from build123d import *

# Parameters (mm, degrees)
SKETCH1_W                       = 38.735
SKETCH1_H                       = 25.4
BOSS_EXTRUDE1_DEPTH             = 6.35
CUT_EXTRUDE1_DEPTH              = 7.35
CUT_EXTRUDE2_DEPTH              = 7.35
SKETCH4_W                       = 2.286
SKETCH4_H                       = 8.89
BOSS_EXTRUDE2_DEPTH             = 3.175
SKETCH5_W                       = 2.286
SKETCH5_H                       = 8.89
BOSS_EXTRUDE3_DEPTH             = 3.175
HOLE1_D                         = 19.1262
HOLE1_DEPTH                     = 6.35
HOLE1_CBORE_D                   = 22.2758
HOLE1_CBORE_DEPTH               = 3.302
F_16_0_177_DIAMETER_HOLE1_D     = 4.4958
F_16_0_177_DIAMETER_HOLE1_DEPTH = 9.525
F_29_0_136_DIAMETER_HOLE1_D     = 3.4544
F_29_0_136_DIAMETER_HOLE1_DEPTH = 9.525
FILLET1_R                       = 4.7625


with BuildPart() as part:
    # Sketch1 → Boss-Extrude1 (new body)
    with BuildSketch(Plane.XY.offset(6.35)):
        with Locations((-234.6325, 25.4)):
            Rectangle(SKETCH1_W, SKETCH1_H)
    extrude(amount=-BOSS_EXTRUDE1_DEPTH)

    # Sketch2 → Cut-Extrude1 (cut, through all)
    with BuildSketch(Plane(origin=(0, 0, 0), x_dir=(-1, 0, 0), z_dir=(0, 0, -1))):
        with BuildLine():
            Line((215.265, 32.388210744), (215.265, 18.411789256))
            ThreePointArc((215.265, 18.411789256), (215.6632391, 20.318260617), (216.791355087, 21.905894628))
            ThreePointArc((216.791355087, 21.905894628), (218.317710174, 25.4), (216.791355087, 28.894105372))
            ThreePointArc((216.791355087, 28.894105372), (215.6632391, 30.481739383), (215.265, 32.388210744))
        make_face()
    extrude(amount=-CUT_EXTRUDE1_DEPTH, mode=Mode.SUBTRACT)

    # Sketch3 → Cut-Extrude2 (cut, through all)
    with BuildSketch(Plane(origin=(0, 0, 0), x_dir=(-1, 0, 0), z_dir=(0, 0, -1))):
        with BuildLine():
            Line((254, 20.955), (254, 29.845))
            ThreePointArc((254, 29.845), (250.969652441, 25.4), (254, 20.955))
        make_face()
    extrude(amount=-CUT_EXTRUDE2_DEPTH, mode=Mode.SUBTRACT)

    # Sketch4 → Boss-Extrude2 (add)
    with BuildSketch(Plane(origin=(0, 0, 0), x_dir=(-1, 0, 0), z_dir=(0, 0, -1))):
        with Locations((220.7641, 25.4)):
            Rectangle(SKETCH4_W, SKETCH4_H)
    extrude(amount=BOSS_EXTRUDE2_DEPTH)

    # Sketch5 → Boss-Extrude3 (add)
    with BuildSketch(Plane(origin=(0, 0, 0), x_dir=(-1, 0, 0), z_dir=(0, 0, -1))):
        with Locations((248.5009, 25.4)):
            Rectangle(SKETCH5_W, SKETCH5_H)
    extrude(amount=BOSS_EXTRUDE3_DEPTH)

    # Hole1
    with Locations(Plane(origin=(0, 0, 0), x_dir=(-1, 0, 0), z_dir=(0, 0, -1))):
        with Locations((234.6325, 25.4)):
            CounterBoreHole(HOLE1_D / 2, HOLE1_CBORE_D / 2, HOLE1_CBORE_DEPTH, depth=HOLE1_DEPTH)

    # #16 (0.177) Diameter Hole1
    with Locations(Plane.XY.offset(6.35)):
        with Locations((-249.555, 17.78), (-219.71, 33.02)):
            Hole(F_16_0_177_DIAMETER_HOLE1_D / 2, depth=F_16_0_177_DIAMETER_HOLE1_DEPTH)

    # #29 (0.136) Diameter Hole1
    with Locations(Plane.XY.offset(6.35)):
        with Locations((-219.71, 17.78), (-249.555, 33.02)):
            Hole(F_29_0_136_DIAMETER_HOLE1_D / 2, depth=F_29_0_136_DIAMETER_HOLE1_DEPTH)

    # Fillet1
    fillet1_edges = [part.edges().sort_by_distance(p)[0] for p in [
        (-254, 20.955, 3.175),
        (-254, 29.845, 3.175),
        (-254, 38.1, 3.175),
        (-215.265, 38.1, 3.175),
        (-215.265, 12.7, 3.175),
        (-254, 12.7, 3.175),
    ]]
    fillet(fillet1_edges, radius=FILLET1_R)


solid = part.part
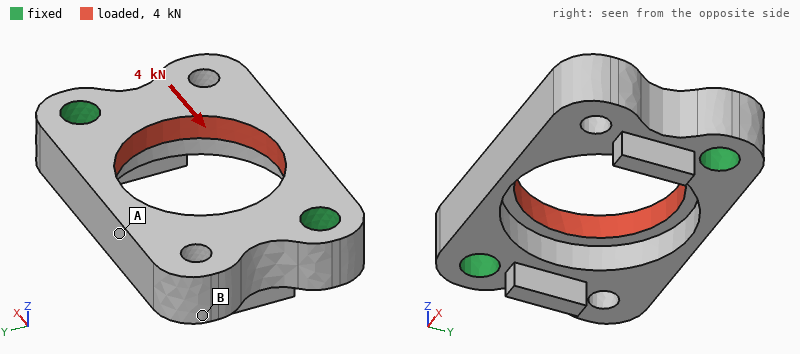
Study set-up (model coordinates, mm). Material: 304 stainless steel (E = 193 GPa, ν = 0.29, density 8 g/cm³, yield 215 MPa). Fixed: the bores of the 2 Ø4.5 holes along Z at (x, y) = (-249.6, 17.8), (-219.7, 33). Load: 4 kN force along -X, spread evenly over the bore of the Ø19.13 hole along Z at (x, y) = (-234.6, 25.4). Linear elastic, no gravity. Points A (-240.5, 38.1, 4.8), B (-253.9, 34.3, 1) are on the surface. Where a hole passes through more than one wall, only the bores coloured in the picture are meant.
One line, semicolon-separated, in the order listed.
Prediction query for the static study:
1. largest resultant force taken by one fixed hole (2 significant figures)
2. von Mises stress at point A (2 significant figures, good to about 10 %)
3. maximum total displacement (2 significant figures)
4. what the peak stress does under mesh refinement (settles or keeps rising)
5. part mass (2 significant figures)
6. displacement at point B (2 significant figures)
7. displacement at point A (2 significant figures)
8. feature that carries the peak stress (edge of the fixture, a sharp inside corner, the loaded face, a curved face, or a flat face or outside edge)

2.0 kN; 39 MPa; 7.1 µm; keeps rising; 28 g; 5.6 µm; 4.8 µm; edge of the fixture
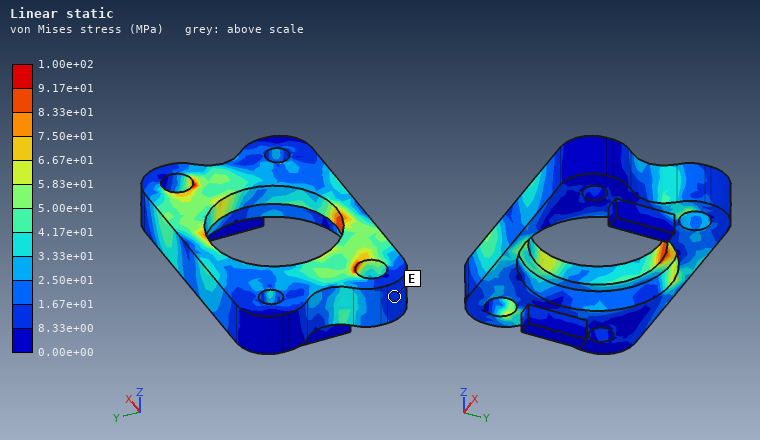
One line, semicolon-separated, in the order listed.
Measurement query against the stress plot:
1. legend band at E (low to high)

8.33e+00 to 1.67e+01 MPa
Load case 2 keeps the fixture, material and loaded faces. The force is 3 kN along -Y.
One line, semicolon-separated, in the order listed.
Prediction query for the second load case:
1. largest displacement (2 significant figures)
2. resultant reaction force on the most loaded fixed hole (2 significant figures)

7.8 µm; 1.5 kN
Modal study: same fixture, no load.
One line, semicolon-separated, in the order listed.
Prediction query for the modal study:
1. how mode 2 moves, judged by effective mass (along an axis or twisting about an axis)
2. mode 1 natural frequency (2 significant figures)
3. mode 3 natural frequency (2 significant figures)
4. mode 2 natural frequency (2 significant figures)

along Z; 13 kHz; 27 kHz; 13 kHz
